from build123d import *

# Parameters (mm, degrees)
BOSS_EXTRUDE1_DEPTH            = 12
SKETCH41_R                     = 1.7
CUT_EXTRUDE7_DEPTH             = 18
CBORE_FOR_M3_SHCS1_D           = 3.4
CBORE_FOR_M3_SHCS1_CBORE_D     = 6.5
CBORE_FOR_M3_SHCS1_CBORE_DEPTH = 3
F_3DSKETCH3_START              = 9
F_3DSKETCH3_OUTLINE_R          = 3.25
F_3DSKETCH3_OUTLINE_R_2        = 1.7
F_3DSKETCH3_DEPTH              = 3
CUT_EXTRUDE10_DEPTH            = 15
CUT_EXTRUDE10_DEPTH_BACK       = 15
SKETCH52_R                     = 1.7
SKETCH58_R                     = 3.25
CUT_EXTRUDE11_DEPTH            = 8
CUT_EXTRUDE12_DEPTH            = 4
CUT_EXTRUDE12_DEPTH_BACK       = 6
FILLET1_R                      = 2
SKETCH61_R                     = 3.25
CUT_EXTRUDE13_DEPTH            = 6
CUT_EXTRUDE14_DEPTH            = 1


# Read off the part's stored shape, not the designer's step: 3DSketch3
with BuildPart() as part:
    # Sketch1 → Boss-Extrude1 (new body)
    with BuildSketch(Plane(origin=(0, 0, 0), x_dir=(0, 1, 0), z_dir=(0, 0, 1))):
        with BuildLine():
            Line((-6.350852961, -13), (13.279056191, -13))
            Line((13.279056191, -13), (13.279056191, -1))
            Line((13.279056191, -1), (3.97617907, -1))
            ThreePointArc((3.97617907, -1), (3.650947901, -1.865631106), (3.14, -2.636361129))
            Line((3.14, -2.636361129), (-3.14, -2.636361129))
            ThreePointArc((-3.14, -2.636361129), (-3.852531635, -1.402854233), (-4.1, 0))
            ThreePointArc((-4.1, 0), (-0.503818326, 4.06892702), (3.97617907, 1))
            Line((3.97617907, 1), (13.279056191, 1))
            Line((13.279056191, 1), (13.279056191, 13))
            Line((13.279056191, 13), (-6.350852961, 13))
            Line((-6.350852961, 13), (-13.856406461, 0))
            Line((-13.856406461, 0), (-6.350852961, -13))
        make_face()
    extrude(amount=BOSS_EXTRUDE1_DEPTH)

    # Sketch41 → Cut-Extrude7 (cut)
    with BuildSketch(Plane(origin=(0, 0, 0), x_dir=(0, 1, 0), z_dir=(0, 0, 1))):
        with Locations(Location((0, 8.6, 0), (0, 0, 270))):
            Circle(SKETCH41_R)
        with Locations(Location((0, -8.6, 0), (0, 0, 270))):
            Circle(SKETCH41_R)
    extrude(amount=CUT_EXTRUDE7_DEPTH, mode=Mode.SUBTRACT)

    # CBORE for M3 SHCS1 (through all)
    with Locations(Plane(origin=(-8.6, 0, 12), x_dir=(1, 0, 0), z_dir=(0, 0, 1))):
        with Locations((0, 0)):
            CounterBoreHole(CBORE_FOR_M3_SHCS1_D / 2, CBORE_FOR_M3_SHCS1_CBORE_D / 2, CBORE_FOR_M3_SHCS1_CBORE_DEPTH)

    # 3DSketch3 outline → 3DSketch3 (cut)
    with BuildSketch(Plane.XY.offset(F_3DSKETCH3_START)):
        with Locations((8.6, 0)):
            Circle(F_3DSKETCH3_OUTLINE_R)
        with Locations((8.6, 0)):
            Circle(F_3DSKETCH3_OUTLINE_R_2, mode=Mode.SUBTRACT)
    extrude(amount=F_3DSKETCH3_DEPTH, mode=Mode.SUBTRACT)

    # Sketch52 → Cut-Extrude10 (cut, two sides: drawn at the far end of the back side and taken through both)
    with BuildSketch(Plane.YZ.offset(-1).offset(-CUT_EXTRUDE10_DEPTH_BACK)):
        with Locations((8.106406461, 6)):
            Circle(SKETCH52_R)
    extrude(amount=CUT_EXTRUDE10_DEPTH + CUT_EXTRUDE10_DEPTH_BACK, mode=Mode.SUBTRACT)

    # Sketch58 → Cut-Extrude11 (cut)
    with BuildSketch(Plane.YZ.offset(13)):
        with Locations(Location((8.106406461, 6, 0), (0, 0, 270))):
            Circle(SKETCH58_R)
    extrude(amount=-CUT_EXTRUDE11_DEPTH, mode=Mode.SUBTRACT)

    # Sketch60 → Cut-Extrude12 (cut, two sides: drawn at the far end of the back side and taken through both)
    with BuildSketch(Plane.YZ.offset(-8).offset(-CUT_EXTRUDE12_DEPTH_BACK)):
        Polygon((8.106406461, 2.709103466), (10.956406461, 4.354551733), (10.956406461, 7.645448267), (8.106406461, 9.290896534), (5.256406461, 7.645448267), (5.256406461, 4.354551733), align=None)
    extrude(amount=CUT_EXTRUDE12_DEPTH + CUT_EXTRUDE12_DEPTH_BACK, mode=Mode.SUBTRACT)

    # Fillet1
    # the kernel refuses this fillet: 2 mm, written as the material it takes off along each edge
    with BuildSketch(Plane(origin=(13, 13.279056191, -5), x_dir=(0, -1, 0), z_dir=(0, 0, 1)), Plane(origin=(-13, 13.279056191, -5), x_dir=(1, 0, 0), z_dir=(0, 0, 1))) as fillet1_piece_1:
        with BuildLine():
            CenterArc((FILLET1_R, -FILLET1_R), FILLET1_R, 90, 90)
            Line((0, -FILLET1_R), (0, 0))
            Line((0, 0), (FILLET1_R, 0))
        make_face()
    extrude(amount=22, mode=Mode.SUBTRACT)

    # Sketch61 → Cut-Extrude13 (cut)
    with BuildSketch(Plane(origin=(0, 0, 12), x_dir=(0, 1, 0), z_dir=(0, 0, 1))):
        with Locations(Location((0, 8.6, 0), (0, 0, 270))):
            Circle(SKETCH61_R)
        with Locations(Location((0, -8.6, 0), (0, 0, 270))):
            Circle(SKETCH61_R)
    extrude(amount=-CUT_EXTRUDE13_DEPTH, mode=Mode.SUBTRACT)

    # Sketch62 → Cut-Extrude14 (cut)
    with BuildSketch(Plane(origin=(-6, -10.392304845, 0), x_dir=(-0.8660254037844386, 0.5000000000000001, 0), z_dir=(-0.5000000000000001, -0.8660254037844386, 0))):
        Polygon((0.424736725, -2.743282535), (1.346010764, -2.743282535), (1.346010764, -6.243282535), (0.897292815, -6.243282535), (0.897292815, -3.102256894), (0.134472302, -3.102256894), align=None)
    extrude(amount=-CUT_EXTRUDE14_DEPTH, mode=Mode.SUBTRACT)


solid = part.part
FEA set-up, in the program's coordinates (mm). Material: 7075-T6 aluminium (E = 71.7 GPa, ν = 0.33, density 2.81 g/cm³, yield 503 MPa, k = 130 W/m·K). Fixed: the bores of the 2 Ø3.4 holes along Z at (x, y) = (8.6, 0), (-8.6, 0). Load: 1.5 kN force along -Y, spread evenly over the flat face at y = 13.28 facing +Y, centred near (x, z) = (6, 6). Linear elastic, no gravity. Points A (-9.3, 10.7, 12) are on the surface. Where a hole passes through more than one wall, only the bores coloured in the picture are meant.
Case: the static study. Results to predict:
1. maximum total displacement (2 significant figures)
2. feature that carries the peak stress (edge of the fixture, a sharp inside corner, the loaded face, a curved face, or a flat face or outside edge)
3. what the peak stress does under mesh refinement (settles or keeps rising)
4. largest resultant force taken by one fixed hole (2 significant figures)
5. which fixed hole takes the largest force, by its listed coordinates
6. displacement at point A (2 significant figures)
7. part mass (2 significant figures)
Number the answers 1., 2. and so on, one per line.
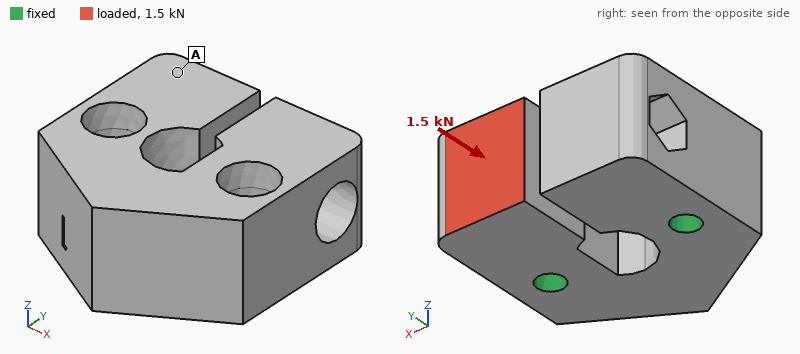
1. 15 µm
2. edge of the fixture
3. keeps rising
4. 1.3 kN
5. (8.6, 0)
6. 2.7 µm
7. 15 g
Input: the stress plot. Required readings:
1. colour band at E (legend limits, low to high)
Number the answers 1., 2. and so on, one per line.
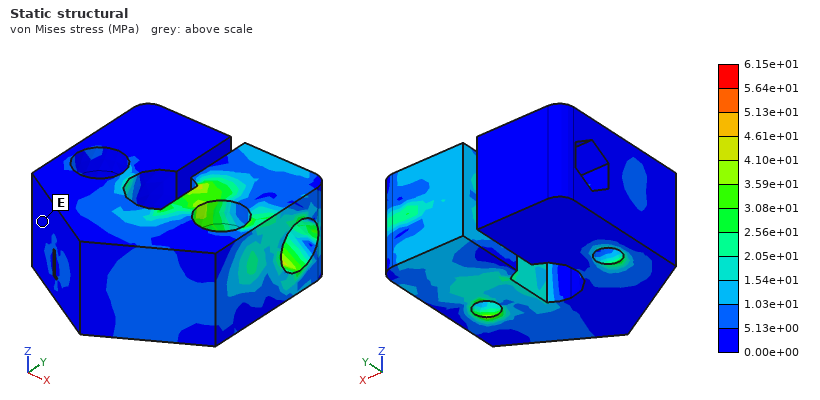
1. 0.00e+00 to 5.13e+00 MPa
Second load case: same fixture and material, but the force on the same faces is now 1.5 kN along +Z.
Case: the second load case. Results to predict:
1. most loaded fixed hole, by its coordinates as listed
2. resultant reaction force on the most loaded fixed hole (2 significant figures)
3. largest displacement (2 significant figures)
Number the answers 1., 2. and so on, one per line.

1. (8.6, 0)
2. 1.6 kN
3. 66 µm
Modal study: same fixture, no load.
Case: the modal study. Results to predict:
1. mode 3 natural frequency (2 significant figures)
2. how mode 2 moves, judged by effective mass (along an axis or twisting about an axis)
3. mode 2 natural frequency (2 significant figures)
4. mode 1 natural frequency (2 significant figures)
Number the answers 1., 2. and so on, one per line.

1. 21 kHz
2. along X
3. 19 kHz
4. 17 kHz
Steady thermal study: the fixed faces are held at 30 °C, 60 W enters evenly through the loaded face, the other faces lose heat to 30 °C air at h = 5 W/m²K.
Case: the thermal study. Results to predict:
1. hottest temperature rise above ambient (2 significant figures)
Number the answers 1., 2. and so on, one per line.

1. 78 K
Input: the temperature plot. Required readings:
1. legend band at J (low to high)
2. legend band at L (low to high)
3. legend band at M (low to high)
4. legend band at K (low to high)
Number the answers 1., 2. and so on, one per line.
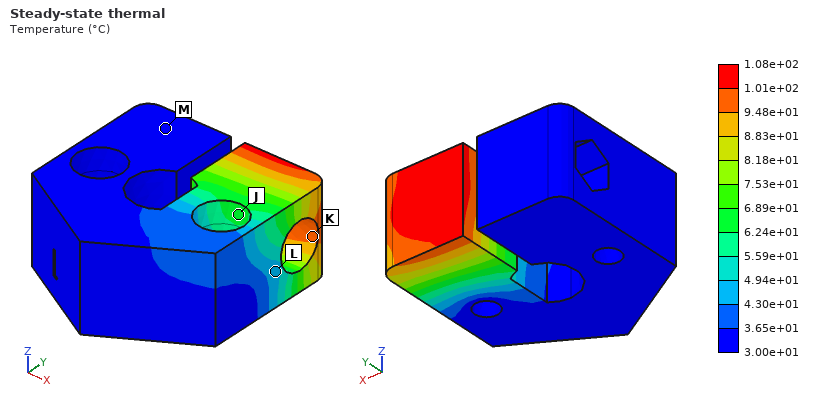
1. 6.24e+01 to 6.89e+01 °C
2. 4.30e+01 to 4.94e+01 °C
3. 3.00e+01 to 3.65e+01 °C
4. 9.48e+01 to 1.01e+02 °C
